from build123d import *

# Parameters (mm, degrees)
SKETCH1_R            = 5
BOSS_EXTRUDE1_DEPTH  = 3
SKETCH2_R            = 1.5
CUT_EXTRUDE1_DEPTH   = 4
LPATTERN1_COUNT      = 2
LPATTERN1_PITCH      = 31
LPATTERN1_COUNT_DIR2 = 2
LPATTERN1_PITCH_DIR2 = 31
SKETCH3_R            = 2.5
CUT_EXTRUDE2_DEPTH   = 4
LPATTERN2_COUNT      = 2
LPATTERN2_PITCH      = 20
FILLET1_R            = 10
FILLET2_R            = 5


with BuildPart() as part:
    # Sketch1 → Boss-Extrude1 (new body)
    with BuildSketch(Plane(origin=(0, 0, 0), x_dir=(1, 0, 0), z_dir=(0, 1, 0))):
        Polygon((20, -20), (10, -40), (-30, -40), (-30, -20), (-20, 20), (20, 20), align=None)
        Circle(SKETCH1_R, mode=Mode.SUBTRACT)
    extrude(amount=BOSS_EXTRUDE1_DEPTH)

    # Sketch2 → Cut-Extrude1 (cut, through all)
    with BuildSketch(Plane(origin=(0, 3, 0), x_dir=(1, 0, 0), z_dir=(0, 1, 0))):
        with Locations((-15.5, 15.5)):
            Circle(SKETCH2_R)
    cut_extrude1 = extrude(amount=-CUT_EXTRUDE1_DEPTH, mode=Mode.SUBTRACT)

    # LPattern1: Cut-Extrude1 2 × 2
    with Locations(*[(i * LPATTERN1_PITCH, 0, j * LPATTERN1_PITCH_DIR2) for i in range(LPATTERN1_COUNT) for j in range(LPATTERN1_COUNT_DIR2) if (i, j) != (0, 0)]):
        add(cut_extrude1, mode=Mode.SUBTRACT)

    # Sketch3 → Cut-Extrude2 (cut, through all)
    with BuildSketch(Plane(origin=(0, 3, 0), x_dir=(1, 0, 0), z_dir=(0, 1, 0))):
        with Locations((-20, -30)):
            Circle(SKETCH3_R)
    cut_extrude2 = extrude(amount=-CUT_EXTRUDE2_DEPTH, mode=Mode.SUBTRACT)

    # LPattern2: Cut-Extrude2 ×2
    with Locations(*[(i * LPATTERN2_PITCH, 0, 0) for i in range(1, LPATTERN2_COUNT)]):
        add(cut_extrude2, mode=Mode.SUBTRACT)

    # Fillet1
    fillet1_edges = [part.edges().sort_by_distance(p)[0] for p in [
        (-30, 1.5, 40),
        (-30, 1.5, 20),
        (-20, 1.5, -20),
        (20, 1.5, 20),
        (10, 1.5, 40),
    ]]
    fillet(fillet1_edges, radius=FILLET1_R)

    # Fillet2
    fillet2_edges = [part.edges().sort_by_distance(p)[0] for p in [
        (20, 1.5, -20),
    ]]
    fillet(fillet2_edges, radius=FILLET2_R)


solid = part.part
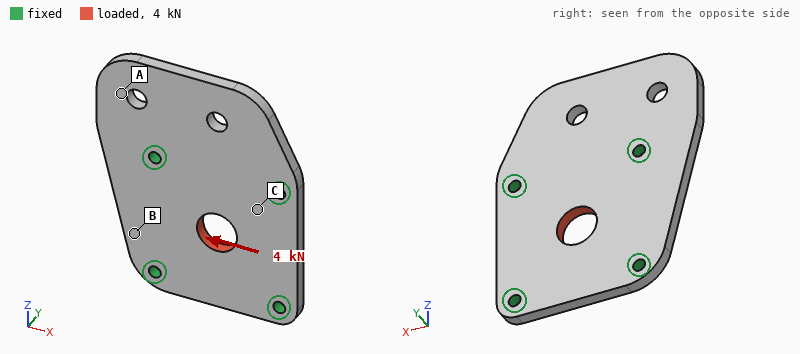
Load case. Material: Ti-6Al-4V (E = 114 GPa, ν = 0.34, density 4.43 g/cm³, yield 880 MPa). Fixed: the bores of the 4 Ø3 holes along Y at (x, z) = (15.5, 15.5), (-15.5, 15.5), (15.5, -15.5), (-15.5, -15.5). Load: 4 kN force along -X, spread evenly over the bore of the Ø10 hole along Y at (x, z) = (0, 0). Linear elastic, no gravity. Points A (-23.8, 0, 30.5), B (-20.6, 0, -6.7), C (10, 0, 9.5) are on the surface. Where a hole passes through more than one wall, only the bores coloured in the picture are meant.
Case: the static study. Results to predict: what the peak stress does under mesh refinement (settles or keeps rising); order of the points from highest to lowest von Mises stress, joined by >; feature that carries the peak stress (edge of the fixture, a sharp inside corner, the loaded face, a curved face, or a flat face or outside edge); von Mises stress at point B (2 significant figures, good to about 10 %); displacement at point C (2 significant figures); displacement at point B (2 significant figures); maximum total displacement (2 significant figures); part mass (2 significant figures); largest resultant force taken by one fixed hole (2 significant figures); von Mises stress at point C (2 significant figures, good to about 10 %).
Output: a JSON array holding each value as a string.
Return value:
["keeps rising", "C > B > A", "edge of the fixture", "16 MPa", "3.4 µm", "3.9 µm", "7.9 µm", "33 g", "1.2 kN", "37 MPa"]
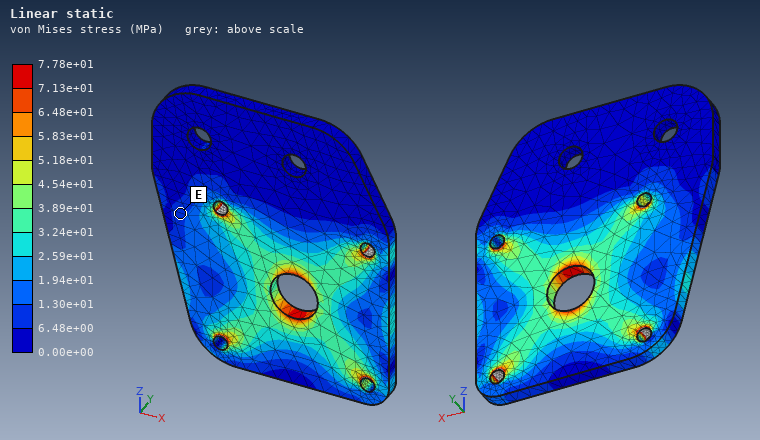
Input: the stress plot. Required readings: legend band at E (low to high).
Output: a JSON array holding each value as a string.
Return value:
["6.48e+00 to 1.30e+01 MPa"]
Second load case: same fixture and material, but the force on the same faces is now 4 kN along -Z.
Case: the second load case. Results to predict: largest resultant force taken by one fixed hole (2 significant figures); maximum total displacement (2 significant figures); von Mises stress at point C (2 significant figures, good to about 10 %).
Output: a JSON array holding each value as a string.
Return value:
["1.2 kN", "7.8 µm", "32 MPa"]
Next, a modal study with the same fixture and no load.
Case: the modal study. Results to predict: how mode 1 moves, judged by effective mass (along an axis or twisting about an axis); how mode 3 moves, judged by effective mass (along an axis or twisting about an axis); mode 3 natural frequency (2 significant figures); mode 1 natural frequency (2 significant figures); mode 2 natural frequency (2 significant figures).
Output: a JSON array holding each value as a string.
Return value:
["along Y", "along Y", "11 kHz", "4000 Hz", "6500 Hz"]
